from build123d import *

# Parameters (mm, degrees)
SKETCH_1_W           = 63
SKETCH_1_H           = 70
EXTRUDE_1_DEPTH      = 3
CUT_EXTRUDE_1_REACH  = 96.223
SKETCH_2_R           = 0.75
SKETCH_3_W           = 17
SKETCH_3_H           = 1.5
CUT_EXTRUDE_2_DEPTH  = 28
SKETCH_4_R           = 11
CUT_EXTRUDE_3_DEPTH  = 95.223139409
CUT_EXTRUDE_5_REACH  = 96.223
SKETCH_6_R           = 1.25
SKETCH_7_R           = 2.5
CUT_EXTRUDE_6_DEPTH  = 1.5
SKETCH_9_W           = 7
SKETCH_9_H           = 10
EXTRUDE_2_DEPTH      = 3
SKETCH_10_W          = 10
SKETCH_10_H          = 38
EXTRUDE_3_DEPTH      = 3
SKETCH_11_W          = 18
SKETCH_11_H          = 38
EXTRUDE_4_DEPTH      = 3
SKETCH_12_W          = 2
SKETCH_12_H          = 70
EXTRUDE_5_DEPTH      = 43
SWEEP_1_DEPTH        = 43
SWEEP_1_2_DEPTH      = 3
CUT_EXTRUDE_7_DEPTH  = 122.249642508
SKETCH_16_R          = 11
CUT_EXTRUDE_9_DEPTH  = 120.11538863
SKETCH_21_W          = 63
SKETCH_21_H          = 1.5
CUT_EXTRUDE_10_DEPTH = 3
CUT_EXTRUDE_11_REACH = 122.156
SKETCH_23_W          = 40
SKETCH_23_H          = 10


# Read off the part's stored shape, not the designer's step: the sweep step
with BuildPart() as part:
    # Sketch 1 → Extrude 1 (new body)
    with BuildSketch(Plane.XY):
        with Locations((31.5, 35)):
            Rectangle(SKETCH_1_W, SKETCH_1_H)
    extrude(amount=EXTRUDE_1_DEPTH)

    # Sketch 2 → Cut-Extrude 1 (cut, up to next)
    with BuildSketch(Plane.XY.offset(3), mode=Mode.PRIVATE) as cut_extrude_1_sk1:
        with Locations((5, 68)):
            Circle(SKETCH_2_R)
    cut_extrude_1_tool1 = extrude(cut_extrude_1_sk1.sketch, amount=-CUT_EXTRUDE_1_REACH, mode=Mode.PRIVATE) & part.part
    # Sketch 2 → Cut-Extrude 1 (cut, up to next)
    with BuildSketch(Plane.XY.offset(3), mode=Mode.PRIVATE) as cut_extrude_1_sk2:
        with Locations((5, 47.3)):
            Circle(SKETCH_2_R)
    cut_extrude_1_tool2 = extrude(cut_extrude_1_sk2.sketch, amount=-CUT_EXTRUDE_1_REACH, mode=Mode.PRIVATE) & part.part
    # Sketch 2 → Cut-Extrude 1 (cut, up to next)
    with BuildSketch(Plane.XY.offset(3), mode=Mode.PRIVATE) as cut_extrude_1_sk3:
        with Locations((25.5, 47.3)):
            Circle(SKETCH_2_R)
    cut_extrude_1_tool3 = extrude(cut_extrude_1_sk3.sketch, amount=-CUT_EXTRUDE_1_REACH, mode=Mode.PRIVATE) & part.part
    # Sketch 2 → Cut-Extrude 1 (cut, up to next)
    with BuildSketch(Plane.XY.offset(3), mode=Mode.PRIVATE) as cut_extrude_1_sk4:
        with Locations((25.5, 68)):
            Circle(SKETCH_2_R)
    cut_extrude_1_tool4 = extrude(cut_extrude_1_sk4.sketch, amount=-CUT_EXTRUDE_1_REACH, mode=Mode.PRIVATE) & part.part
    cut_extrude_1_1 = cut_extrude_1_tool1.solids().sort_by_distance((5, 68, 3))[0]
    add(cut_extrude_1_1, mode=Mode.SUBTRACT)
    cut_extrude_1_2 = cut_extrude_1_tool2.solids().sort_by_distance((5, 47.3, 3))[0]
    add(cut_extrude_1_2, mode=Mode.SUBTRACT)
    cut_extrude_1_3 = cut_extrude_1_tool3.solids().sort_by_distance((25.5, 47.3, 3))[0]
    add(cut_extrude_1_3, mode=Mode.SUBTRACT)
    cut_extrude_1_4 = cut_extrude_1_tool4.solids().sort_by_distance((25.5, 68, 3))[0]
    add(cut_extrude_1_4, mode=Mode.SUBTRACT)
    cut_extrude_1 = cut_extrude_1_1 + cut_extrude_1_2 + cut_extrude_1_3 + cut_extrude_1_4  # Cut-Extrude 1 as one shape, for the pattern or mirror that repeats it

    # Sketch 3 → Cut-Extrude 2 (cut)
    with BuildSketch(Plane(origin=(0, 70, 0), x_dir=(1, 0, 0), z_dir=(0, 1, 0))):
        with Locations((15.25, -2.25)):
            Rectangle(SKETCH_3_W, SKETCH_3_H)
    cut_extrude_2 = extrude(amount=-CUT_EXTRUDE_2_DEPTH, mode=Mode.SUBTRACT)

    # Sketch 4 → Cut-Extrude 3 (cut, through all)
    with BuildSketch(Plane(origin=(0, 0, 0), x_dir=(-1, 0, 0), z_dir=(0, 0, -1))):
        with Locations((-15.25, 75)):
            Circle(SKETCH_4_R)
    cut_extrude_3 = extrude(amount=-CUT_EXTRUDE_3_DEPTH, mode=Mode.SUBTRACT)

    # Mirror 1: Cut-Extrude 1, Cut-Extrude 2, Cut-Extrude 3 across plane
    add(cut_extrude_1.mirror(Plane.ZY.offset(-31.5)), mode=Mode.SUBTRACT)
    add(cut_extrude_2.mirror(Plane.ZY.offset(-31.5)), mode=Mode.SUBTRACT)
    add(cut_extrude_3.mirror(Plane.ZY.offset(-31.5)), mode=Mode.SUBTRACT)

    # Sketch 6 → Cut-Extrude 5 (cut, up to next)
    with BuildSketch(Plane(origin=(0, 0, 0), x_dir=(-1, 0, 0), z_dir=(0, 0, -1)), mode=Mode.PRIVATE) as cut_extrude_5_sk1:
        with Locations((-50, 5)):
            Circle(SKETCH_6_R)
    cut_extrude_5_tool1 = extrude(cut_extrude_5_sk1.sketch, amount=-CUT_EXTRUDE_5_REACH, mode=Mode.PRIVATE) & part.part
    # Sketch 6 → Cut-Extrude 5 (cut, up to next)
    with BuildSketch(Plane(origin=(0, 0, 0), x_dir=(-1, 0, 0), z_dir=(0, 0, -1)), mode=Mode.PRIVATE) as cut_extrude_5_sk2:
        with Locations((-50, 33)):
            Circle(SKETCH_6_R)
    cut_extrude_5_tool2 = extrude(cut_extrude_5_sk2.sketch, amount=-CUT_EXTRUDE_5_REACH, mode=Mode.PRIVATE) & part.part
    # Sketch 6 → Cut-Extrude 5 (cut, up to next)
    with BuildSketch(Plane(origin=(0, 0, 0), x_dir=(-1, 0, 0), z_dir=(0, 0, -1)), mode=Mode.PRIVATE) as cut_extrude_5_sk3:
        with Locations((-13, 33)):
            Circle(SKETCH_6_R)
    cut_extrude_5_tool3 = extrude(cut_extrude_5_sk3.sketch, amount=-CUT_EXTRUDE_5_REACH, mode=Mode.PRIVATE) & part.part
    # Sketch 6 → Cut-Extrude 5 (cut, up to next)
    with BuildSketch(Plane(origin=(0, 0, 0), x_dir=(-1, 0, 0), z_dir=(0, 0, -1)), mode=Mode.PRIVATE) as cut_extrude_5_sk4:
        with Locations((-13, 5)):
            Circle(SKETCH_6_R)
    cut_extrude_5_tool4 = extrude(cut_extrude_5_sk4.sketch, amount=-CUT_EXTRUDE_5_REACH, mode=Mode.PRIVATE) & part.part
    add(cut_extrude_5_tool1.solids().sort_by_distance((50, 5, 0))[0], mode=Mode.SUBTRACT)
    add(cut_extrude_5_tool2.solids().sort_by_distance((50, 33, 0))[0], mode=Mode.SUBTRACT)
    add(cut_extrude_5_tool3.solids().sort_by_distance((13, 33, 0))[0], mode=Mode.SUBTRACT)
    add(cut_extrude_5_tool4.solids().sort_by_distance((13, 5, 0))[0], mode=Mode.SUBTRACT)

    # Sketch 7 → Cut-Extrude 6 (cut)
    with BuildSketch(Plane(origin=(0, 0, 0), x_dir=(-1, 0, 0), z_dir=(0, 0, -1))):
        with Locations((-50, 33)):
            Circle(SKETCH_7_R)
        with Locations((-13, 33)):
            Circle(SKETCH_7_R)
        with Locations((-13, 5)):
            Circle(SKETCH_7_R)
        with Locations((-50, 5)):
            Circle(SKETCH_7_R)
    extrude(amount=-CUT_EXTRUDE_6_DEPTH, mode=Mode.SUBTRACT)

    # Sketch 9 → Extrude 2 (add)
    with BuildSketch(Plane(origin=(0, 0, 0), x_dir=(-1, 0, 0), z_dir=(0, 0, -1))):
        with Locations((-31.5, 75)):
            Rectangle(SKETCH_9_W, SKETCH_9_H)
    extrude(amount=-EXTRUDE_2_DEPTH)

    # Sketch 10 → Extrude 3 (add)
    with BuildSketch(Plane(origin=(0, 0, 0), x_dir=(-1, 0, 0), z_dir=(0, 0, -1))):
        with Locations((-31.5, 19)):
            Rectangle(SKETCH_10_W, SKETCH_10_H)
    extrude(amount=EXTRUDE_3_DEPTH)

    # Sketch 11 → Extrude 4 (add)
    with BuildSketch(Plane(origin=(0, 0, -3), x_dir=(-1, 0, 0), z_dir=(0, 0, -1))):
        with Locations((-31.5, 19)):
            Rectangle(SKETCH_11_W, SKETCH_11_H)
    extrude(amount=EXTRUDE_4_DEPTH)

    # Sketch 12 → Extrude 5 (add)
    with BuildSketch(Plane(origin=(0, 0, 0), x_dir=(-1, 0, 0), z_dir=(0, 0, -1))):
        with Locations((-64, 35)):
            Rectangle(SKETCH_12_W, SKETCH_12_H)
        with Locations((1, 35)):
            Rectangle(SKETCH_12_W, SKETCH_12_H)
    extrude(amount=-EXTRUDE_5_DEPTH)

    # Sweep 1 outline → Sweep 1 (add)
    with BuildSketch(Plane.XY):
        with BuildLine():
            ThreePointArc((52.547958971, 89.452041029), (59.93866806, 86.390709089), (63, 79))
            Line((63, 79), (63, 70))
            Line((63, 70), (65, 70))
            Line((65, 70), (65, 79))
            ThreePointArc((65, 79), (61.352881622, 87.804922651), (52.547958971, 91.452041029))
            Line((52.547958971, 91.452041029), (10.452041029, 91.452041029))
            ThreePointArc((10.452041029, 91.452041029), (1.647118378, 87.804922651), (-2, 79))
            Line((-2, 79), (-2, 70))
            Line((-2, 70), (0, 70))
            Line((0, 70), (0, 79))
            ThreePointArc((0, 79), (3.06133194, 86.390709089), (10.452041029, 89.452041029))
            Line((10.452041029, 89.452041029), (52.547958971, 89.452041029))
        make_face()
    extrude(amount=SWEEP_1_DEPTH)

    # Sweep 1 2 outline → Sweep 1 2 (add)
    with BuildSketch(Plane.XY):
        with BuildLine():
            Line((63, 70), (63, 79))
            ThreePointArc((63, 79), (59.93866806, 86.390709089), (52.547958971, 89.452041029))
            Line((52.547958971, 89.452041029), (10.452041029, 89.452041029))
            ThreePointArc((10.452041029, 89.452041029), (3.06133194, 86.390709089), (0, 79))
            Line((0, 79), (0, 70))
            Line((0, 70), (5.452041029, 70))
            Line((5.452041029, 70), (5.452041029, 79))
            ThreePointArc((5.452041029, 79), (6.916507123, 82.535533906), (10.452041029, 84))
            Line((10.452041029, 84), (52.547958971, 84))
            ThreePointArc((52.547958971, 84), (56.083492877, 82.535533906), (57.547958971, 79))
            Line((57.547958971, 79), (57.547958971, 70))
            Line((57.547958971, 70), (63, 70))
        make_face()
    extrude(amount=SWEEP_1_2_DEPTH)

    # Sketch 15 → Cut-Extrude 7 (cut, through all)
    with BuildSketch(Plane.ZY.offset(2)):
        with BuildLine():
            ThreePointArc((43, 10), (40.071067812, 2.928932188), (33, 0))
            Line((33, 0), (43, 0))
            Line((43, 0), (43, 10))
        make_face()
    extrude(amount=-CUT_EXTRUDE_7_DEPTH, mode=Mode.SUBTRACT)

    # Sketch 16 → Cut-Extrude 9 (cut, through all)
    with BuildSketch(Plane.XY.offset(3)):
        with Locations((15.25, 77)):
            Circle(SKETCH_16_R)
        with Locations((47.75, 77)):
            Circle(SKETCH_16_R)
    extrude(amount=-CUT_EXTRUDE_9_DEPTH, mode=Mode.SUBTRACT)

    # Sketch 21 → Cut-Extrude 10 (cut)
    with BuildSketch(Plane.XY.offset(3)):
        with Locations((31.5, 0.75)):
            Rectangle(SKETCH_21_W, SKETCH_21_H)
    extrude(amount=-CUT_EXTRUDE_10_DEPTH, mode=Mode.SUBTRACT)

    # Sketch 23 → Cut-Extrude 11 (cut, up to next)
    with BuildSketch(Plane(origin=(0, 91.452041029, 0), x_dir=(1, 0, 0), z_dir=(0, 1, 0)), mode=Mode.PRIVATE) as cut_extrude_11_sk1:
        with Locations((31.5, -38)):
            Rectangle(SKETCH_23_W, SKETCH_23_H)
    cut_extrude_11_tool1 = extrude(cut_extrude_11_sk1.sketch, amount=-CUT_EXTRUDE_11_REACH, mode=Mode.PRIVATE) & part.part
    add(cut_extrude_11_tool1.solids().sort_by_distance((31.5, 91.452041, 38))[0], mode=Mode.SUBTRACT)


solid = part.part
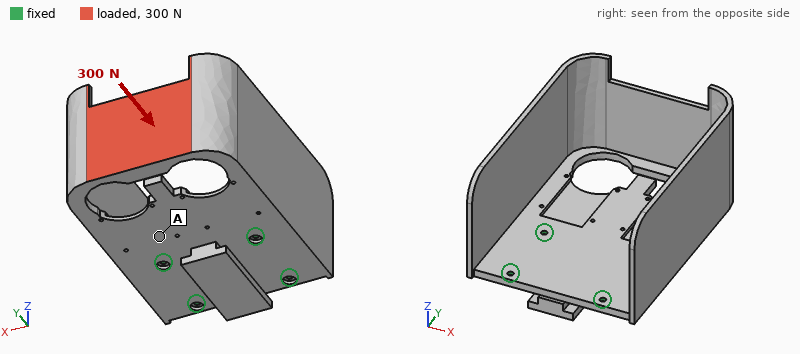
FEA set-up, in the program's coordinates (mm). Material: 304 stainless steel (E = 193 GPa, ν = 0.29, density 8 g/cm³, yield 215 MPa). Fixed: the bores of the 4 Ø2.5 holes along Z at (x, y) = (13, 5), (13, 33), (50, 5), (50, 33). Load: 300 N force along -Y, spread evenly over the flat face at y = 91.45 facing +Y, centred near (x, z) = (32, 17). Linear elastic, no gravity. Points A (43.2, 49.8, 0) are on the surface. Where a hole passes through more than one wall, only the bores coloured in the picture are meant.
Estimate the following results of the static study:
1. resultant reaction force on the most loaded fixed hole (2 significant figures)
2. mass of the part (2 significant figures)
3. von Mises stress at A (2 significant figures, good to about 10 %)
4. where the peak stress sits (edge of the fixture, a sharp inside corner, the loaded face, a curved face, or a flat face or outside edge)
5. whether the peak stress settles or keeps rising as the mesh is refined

160 N
280 g
6.7 MPa
edge of the fixture
keeps rising
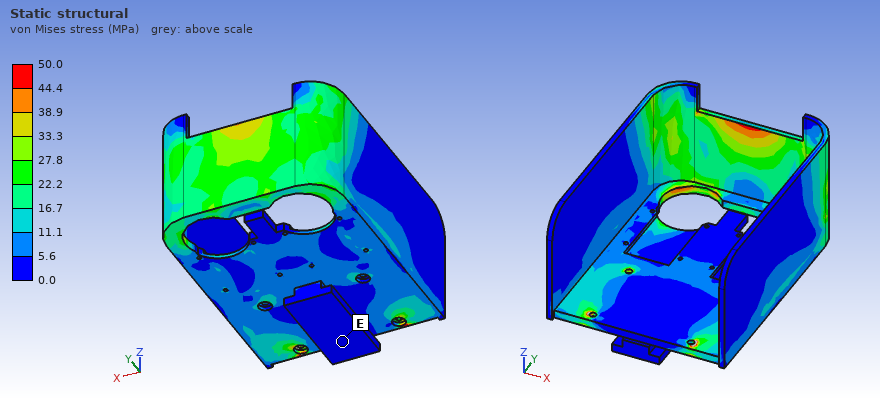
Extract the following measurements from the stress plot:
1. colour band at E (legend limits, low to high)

0.0 to 5.6 MPa
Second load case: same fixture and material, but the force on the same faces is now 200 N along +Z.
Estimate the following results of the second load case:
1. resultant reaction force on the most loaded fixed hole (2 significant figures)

370 N
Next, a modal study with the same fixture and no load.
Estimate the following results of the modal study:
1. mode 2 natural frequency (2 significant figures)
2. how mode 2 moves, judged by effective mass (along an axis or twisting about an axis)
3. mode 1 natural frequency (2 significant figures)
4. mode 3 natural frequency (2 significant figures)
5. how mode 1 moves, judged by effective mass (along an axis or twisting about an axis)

750 Hz
along Z
640 Hz
920 Hz
along X
